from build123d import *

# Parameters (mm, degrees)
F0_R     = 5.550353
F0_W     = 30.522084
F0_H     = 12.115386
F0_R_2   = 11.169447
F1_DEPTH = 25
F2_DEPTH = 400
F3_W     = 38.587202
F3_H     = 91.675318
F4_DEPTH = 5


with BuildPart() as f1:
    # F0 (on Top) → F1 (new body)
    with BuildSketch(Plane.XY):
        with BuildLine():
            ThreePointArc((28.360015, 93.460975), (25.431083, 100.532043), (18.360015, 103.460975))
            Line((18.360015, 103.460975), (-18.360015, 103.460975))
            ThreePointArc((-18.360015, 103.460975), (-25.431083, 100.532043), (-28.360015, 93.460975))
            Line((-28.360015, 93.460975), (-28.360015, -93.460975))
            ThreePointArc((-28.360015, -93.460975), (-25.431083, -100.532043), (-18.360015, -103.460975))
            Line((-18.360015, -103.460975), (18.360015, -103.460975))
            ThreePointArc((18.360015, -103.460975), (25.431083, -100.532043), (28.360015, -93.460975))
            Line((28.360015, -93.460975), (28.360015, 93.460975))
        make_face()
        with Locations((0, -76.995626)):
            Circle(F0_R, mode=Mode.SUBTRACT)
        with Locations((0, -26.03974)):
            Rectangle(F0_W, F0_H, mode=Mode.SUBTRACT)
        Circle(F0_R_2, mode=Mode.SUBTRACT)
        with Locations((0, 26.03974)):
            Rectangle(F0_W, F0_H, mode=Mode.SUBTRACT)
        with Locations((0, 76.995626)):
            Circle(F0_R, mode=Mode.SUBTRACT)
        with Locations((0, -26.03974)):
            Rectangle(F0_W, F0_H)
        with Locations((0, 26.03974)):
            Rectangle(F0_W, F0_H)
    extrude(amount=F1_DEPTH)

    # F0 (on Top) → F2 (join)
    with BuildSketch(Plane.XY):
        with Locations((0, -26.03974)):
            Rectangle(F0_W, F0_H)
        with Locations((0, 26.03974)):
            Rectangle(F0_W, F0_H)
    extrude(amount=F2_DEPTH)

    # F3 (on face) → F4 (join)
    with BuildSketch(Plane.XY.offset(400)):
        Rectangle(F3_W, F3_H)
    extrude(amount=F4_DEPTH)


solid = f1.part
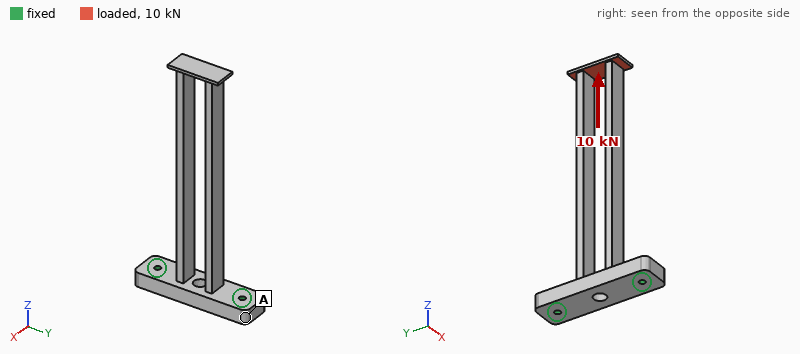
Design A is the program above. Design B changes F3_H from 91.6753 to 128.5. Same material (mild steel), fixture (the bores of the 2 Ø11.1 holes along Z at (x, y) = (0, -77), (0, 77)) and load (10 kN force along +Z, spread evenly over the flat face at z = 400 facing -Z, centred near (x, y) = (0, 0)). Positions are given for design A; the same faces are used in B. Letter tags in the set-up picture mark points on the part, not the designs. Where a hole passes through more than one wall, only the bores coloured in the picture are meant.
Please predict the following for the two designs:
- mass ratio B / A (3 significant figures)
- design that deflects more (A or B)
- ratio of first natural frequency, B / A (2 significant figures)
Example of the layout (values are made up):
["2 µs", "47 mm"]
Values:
["1.01", "B", "0.97"]
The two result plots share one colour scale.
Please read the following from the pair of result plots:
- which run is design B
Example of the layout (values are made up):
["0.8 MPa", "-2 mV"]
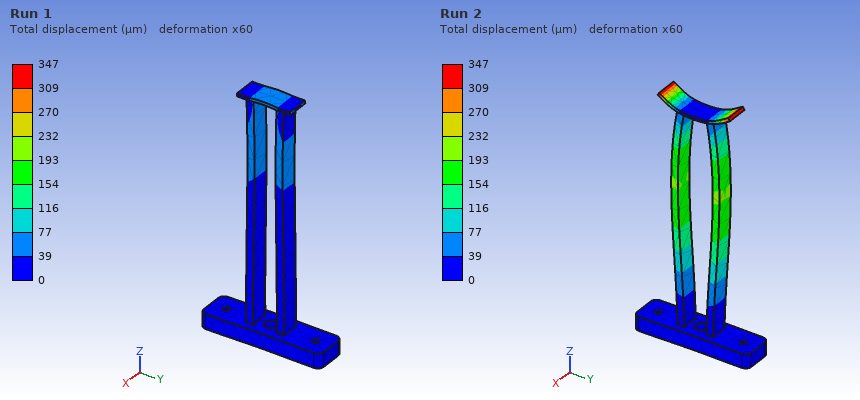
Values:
["Run 2"]
